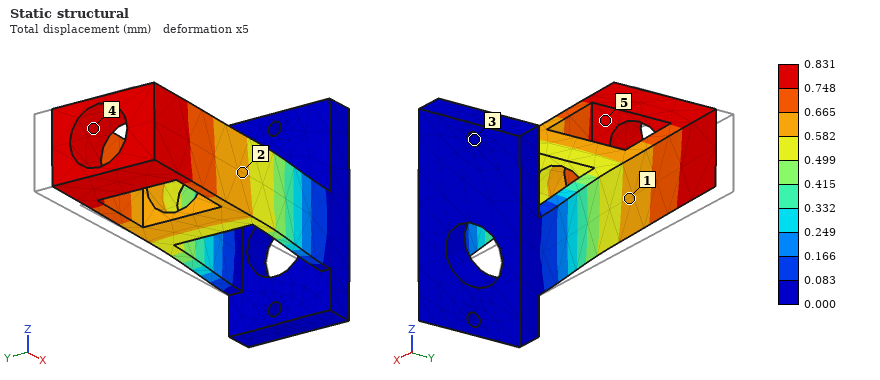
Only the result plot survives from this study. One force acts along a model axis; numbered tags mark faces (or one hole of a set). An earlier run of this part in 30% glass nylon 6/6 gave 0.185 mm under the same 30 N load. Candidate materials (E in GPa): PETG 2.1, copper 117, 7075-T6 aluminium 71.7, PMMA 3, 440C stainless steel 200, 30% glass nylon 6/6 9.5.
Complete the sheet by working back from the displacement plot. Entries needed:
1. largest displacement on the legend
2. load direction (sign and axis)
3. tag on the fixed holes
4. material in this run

0.831 mm
-Y
3
PETG
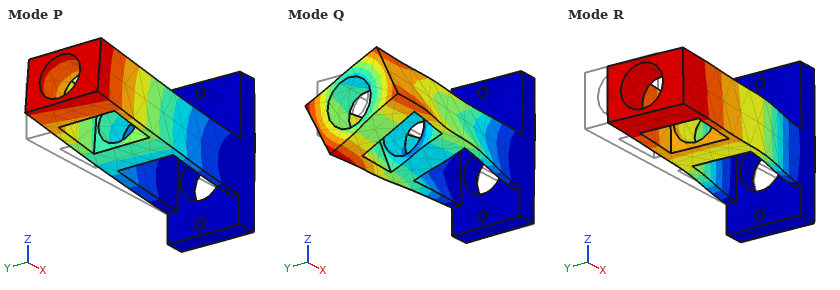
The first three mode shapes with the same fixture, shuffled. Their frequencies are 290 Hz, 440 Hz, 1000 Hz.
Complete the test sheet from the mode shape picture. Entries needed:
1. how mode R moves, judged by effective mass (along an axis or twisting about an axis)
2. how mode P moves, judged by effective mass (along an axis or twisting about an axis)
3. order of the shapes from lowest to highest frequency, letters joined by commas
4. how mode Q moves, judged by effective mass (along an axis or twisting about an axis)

along Y
along Z
R, P, Q
twisting about X
